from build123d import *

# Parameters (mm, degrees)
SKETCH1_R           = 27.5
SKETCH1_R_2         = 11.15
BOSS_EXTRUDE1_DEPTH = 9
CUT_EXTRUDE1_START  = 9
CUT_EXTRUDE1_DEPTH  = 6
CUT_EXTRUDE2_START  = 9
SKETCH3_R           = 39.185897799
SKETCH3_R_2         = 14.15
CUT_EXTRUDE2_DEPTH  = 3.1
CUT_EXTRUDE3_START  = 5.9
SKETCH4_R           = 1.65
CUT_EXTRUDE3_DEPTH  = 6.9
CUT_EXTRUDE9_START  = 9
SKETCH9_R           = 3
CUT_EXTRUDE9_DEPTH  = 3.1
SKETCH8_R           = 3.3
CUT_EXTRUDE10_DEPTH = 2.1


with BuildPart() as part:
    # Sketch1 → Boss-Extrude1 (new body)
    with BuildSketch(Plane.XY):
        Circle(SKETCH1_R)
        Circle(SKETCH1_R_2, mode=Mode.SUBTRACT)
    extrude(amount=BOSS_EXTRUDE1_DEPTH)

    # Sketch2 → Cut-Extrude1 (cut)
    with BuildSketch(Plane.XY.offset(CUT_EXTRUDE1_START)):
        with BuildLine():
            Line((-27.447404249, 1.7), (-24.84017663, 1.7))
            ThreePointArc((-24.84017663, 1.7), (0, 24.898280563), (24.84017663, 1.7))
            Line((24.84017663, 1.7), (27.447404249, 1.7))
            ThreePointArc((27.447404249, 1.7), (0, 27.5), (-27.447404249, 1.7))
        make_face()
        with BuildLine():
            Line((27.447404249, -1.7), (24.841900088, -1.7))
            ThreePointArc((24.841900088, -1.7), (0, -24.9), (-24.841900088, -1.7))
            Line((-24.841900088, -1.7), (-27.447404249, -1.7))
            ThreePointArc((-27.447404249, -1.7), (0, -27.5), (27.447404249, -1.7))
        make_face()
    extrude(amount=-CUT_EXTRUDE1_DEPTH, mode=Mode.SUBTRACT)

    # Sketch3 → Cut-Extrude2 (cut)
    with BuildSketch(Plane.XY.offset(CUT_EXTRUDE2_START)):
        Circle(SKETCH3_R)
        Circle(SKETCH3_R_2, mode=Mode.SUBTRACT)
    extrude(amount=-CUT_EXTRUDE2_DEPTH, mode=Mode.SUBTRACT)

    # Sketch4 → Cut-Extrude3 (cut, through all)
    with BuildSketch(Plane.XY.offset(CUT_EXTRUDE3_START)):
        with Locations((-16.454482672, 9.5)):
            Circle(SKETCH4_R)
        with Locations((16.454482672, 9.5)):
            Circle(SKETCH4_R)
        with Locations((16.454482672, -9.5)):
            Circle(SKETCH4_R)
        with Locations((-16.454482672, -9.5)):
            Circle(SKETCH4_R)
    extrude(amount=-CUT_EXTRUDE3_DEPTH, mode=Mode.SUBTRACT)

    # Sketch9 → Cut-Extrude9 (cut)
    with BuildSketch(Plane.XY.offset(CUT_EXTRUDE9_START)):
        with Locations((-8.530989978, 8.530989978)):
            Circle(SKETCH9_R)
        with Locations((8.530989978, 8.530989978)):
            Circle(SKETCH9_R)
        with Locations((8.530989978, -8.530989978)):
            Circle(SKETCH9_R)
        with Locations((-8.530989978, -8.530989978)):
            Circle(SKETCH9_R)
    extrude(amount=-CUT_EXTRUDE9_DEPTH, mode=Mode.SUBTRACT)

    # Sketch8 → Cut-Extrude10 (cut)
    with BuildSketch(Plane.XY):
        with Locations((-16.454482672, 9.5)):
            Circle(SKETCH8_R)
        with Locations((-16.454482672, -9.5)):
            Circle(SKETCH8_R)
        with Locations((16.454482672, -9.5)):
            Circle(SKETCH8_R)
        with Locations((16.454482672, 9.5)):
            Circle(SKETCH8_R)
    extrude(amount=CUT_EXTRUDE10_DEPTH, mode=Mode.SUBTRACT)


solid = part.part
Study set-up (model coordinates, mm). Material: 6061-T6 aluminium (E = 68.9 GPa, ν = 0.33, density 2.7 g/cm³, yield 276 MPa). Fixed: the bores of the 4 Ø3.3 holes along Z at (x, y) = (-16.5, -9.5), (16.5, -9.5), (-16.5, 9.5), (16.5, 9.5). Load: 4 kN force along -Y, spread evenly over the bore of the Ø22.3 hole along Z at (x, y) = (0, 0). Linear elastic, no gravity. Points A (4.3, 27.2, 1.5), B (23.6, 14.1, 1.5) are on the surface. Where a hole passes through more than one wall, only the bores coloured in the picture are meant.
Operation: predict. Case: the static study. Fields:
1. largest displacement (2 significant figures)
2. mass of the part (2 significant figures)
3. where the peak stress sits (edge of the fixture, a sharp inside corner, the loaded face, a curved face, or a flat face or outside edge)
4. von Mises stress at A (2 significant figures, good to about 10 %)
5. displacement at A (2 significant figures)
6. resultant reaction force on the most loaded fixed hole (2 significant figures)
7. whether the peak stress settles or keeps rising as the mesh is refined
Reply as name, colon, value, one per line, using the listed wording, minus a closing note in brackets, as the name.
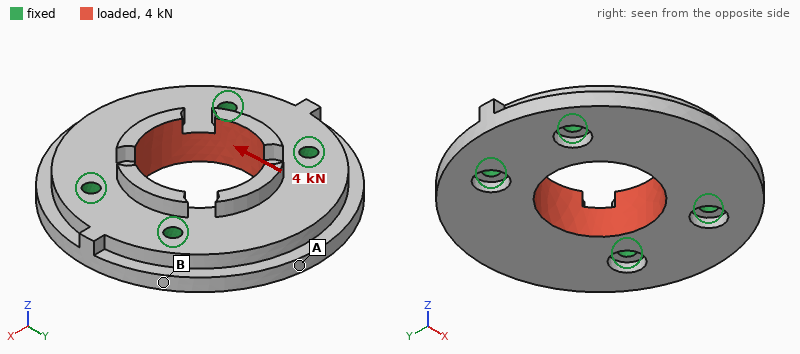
largest displacement: 9.2 µm
mass of the part: 29 g
where the peak stress sits: edge of the fixture
von Mises stress at A: 11 MPa
displacement at A: 4.2 µm
resultant reaction force on the most loaded fixed hole: 1.0 kN
whether the peak stress settles or keeps rising as the mesh is refined: keeps rising
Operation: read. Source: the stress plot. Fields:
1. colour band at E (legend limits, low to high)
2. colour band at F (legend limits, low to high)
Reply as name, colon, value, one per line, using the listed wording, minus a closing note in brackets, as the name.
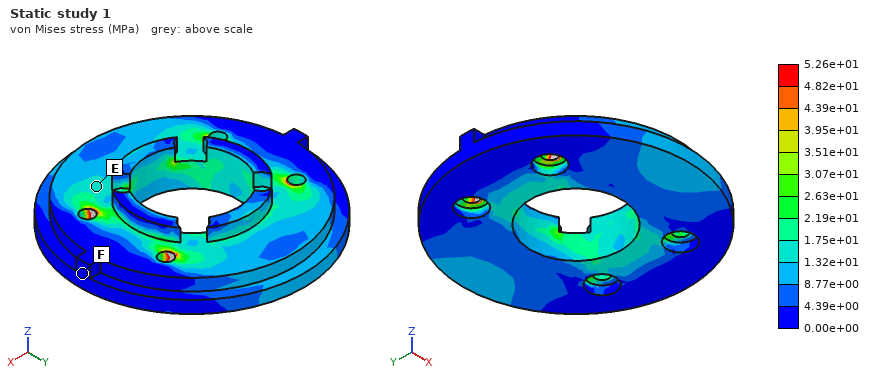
colour band at E: 1.32e+01 to 1.75e+01 MPa
colour band at F: 0.00e+00 to 4.39e+00 MPa
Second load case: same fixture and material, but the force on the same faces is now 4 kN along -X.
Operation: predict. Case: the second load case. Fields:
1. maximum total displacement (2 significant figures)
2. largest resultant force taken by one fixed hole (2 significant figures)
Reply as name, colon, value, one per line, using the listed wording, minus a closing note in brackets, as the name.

maximum total displacement: 5.2 µm
largest resultant force taken by one fixed hole: 1.0 kN
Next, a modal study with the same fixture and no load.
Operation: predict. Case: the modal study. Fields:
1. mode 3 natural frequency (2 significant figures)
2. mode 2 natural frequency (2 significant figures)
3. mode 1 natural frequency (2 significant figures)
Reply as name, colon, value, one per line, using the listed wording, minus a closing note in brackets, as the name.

mode 3 natural frequency: 25 kHz
mode 2 natural frequency: 11 kHz
mode 1 natural frequency: 11 kHz
